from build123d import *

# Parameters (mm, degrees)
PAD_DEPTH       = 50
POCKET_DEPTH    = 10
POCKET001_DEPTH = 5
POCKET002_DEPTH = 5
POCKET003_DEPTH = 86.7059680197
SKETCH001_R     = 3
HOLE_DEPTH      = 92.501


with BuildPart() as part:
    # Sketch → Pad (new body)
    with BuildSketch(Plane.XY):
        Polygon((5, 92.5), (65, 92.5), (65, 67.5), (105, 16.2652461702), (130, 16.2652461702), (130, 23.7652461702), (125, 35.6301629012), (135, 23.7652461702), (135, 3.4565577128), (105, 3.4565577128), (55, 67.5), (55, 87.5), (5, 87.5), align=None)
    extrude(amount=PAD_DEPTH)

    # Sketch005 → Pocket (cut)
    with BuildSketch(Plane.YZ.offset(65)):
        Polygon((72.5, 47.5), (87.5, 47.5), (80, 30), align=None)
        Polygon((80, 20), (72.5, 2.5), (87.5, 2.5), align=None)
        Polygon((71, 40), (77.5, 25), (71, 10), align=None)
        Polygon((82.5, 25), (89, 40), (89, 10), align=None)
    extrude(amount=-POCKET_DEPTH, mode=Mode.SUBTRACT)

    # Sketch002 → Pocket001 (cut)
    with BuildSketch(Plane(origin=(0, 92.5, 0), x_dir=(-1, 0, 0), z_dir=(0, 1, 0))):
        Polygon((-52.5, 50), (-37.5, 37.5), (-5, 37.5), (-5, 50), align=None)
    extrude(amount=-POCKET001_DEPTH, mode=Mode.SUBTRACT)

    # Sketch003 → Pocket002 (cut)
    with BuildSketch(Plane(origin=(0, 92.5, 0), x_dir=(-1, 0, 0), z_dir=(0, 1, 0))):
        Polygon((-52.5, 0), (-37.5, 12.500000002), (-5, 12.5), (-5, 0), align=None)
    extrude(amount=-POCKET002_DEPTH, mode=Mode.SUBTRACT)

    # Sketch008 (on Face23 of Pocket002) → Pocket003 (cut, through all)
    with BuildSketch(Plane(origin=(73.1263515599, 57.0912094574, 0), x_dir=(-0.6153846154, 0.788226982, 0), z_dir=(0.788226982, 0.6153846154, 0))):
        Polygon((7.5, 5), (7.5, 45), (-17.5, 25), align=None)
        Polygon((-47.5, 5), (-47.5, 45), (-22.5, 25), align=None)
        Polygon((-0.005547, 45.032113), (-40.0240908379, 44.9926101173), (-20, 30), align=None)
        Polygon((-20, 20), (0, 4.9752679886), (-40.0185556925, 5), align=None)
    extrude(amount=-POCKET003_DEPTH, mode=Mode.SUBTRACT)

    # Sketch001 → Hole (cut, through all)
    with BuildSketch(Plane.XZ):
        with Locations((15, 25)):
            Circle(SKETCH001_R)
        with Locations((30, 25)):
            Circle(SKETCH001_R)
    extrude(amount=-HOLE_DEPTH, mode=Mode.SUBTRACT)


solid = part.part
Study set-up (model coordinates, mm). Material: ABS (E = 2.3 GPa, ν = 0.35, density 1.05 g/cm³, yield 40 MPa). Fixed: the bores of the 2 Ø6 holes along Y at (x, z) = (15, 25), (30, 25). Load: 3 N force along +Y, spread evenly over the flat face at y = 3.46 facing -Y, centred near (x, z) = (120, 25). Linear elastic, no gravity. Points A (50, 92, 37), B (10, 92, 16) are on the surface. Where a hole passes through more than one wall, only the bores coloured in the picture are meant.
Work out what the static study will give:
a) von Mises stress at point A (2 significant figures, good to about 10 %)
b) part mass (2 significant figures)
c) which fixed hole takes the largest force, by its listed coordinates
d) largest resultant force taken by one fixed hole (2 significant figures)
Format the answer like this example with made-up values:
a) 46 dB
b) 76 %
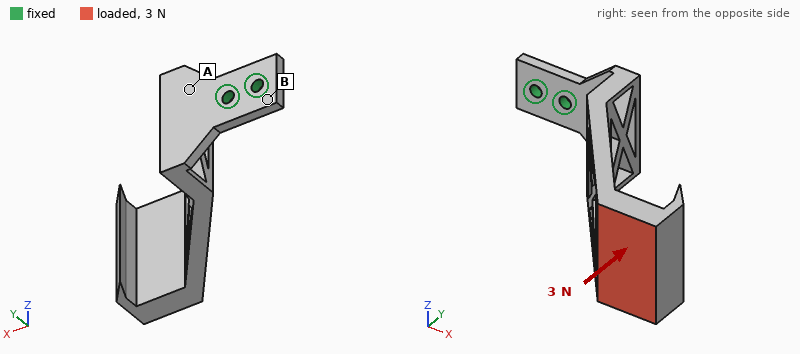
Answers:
a) 1.2 MPa
b) 57 g
c) (30, 25)
d) 7.4 N
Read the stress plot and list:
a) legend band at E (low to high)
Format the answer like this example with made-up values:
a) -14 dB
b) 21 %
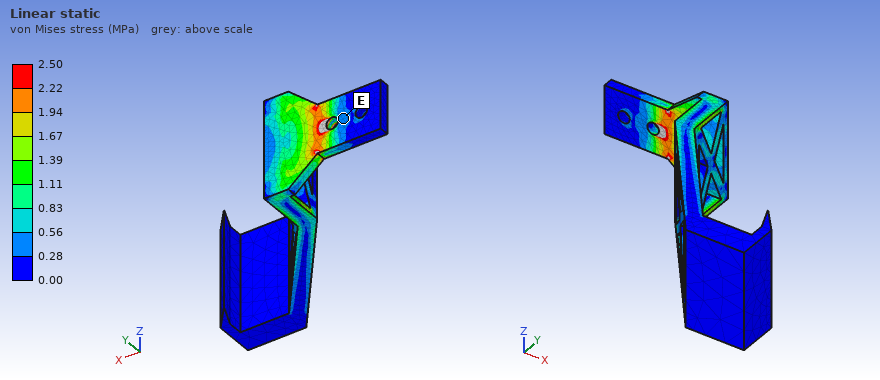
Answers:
a) 0.28 to 0.56 MPa
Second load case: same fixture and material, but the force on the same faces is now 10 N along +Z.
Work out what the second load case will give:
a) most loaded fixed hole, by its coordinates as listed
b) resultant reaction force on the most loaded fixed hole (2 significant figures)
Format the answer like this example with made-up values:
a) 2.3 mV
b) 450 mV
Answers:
a) (30, 25)
b) 44 N
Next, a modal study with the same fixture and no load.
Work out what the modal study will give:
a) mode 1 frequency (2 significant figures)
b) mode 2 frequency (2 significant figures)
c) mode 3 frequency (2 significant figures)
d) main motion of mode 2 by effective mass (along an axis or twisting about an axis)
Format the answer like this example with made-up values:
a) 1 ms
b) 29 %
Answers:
a) 34 Hz
b) 71 Hz
c) 230 Hz
d) along Z
